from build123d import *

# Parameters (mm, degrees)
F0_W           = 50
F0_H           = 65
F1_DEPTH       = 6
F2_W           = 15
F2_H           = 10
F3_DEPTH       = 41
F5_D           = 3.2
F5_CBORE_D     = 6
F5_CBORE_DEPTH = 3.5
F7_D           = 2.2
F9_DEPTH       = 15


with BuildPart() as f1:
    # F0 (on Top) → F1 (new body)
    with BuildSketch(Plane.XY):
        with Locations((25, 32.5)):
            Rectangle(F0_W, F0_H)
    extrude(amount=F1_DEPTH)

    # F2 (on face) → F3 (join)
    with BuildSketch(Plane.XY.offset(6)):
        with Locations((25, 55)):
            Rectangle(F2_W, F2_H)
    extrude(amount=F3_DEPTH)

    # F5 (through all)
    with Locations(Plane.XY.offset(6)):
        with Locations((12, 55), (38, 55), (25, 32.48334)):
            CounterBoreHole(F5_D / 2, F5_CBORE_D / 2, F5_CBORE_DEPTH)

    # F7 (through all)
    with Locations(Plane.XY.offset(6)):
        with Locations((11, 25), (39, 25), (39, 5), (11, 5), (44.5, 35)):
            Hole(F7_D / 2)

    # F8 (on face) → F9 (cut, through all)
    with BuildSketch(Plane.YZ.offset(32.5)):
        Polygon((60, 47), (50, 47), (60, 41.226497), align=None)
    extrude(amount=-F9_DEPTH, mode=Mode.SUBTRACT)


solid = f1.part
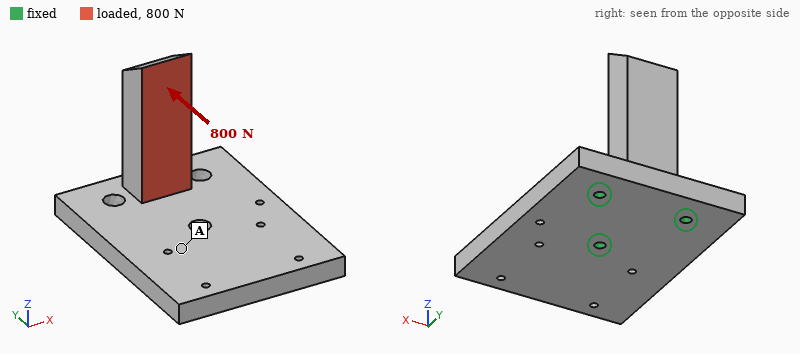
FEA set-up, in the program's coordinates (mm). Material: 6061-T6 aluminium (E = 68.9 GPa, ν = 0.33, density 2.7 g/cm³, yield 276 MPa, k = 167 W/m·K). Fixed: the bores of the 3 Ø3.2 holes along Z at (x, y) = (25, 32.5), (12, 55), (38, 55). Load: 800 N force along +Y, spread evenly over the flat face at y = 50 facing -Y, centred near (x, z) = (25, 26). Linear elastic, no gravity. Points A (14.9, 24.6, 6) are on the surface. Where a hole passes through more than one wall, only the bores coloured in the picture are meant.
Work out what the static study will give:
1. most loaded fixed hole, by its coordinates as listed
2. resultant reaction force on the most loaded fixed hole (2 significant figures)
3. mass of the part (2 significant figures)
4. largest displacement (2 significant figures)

(25, 32.5)
1.2 kN
67 g
0.19 mm
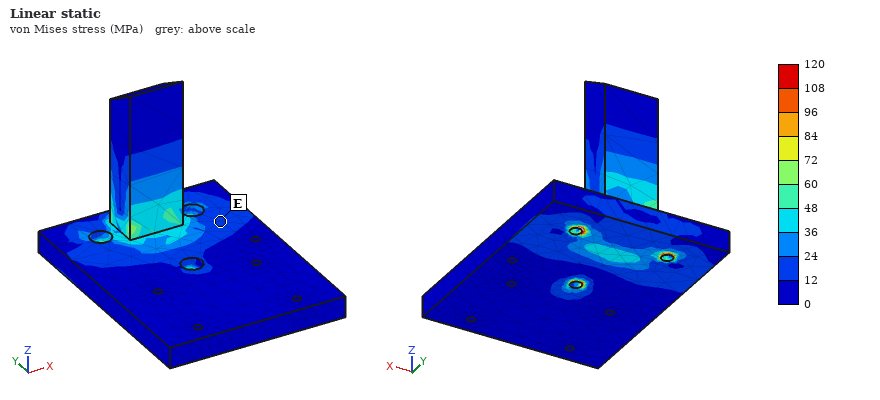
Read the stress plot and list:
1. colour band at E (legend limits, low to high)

12 to 24 MPa
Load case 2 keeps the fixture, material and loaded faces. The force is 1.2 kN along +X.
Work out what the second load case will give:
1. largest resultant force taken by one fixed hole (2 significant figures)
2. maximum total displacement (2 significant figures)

1.3 kN
0.12 mm
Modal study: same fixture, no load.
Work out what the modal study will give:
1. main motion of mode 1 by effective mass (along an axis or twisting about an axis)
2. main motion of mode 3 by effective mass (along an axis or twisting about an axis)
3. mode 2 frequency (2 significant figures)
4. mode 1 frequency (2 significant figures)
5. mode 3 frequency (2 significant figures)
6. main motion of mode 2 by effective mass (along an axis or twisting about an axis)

along Z
twisting about Y
3500 Hz
3200 Hz
3900 Hz
along Y
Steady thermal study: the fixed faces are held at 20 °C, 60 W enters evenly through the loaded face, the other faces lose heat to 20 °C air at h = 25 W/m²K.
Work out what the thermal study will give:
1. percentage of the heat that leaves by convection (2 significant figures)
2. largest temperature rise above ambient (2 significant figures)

5.5 %
72 K
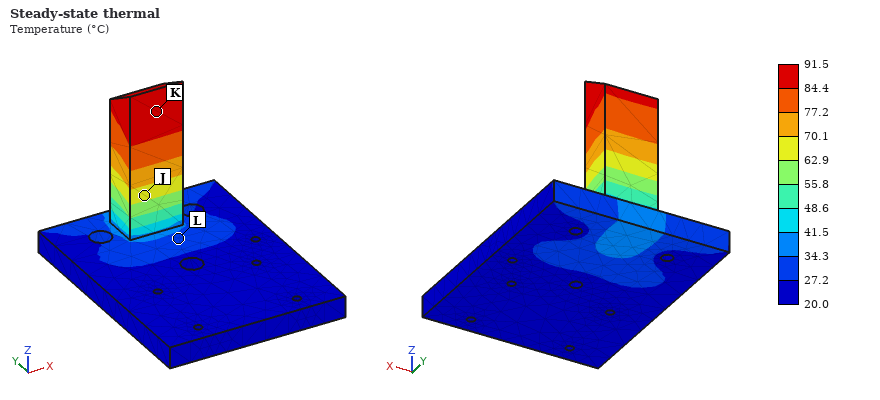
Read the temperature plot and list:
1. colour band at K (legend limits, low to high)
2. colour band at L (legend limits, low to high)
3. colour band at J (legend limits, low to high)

84.4 to 91.5 °C
27.2 to 34.3 °C
62.9 to 70.1 °C
